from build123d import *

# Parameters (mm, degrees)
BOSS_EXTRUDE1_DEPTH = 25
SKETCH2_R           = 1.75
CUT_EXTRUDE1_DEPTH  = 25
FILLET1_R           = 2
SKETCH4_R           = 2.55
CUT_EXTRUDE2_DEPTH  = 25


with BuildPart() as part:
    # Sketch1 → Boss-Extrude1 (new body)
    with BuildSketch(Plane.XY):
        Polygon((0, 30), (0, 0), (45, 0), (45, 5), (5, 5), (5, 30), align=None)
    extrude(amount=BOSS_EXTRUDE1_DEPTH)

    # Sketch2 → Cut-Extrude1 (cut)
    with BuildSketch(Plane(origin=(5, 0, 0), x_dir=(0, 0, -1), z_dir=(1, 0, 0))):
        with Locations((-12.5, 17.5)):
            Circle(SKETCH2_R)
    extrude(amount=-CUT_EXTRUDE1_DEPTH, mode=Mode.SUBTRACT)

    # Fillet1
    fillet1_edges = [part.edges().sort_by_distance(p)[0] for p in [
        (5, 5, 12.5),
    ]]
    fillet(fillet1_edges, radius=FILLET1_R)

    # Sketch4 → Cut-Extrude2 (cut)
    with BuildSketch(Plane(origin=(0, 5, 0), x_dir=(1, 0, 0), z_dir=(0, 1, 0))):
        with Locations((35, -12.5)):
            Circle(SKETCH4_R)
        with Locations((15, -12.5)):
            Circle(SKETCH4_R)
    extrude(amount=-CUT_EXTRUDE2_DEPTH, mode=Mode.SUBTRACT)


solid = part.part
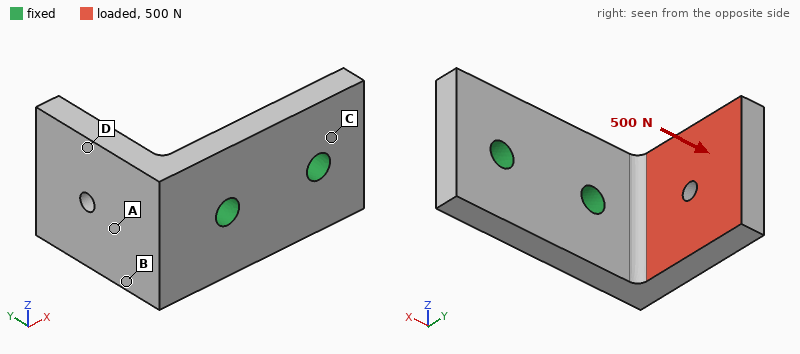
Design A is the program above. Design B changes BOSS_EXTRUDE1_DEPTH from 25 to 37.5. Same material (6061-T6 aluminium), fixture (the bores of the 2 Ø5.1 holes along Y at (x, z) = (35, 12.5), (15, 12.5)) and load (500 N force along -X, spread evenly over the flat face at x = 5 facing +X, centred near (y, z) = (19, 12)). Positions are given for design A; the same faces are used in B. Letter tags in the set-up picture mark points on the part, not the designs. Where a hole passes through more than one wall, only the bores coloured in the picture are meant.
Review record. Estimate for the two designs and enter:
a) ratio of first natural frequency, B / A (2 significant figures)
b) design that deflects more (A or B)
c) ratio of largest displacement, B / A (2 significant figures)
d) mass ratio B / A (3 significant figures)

0.91
A
0.75
1.51
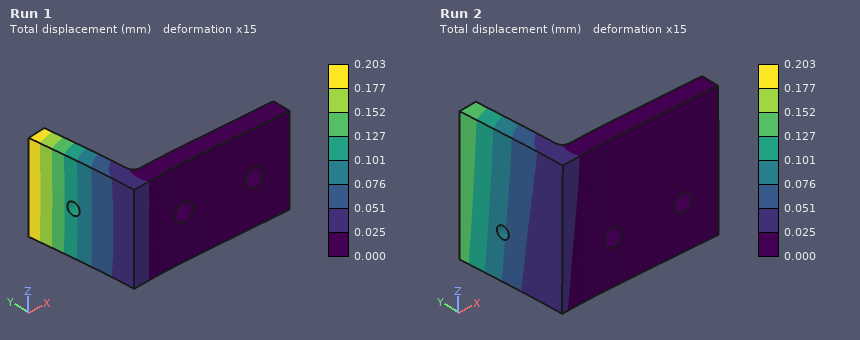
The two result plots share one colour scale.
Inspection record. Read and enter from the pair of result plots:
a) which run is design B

Run 2
